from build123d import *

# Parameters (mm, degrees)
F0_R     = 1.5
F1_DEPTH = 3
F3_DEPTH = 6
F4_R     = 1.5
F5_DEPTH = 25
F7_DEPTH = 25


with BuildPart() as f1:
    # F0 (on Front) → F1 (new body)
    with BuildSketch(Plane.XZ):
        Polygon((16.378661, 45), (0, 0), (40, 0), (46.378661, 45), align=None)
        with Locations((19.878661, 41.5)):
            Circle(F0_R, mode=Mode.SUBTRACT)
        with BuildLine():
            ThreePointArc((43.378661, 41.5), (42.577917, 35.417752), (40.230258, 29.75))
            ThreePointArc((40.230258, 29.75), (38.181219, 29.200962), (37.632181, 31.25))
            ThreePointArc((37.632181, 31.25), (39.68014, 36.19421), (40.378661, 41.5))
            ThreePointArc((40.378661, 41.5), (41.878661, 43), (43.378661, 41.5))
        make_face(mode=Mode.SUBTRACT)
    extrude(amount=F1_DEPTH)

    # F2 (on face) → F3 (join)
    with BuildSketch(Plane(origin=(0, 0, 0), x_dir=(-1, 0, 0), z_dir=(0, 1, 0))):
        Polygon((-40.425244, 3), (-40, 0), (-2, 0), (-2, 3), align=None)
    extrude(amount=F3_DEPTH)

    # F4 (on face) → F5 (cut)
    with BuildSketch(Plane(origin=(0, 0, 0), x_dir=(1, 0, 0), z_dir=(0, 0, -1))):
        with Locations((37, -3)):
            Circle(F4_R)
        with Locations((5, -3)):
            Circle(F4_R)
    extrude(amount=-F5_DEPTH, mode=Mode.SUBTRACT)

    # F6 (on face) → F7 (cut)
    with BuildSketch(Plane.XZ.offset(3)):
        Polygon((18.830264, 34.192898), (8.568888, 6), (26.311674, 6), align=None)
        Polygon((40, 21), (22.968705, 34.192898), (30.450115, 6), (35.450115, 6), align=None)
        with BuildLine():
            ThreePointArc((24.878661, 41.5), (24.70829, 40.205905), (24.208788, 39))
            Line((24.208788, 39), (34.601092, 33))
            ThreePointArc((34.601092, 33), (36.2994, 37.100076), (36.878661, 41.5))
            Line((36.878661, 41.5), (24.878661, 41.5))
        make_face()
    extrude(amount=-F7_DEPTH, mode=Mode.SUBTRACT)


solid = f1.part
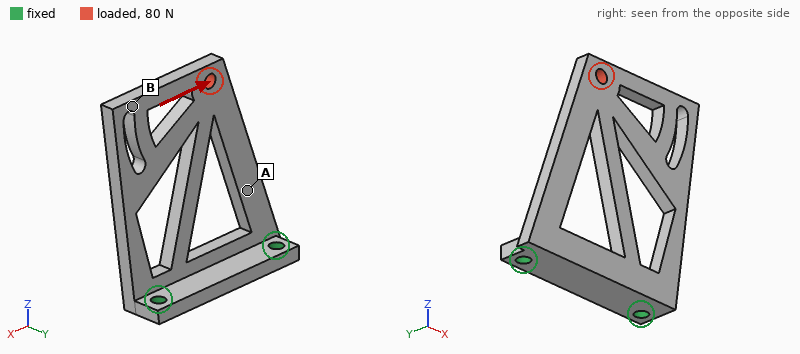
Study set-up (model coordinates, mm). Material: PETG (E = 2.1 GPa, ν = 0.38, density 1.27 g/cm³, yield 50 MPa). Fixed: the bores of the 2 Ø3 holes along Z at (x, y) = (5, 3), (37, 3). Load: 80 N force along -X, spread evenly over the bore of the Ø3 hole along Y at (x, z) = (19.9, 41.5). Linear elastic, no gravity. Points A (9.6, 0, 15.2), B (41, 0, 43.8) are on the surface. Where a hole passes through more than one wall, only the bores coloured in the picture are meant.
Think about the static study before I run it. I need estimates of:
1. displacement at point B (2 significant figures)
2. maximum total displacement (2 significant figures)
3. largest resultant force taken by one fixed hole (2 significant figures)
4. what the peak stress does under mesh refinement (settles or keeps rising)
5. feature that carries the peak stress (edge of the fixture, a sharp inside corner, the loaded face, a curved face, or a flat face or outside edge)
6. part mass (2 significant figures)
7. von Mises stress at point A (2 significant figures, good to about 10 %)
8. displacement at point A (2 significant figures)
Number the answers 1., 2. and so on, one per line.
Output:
1. 0.70 mm
2. 0.74 mm
3. 110 N
4. keeps rising
5. edge of the fixture
6. 4.5 g
7. 7.6 MPa
8. 0.23 mm
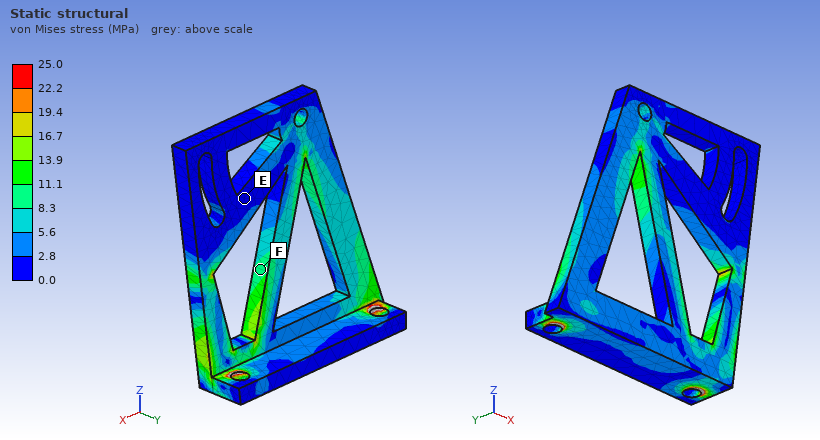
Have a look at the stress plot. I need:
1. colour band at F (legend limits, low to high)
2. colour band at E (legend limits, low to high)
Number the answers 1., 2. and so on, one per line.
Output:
1. 8.3 to 11.1 MPa
2. 0.0 to 2.8 MPa
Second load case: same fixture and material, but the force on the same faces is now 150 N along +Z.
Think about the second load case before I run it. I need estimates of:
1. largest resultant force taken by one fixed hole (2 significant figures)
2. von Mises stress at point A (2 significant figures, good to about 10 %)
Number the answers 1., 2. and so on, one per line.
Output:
1. 80 N
2. 4.3 MPa
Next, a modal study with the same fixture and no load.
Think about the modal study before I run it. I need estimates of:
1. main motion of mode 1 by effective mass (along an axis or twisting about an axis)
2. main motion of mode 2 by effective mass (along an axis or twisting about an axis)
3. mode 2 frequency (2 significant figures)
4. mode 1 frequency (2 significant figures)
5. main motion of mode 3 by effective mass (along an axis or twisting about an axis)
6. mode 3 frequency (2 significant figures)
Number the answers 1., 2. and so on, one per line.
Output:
1. along Y
2. twisting about Z
3. 720 Hz
4. 250 Hz
5. along X
6. 1400 Hz
